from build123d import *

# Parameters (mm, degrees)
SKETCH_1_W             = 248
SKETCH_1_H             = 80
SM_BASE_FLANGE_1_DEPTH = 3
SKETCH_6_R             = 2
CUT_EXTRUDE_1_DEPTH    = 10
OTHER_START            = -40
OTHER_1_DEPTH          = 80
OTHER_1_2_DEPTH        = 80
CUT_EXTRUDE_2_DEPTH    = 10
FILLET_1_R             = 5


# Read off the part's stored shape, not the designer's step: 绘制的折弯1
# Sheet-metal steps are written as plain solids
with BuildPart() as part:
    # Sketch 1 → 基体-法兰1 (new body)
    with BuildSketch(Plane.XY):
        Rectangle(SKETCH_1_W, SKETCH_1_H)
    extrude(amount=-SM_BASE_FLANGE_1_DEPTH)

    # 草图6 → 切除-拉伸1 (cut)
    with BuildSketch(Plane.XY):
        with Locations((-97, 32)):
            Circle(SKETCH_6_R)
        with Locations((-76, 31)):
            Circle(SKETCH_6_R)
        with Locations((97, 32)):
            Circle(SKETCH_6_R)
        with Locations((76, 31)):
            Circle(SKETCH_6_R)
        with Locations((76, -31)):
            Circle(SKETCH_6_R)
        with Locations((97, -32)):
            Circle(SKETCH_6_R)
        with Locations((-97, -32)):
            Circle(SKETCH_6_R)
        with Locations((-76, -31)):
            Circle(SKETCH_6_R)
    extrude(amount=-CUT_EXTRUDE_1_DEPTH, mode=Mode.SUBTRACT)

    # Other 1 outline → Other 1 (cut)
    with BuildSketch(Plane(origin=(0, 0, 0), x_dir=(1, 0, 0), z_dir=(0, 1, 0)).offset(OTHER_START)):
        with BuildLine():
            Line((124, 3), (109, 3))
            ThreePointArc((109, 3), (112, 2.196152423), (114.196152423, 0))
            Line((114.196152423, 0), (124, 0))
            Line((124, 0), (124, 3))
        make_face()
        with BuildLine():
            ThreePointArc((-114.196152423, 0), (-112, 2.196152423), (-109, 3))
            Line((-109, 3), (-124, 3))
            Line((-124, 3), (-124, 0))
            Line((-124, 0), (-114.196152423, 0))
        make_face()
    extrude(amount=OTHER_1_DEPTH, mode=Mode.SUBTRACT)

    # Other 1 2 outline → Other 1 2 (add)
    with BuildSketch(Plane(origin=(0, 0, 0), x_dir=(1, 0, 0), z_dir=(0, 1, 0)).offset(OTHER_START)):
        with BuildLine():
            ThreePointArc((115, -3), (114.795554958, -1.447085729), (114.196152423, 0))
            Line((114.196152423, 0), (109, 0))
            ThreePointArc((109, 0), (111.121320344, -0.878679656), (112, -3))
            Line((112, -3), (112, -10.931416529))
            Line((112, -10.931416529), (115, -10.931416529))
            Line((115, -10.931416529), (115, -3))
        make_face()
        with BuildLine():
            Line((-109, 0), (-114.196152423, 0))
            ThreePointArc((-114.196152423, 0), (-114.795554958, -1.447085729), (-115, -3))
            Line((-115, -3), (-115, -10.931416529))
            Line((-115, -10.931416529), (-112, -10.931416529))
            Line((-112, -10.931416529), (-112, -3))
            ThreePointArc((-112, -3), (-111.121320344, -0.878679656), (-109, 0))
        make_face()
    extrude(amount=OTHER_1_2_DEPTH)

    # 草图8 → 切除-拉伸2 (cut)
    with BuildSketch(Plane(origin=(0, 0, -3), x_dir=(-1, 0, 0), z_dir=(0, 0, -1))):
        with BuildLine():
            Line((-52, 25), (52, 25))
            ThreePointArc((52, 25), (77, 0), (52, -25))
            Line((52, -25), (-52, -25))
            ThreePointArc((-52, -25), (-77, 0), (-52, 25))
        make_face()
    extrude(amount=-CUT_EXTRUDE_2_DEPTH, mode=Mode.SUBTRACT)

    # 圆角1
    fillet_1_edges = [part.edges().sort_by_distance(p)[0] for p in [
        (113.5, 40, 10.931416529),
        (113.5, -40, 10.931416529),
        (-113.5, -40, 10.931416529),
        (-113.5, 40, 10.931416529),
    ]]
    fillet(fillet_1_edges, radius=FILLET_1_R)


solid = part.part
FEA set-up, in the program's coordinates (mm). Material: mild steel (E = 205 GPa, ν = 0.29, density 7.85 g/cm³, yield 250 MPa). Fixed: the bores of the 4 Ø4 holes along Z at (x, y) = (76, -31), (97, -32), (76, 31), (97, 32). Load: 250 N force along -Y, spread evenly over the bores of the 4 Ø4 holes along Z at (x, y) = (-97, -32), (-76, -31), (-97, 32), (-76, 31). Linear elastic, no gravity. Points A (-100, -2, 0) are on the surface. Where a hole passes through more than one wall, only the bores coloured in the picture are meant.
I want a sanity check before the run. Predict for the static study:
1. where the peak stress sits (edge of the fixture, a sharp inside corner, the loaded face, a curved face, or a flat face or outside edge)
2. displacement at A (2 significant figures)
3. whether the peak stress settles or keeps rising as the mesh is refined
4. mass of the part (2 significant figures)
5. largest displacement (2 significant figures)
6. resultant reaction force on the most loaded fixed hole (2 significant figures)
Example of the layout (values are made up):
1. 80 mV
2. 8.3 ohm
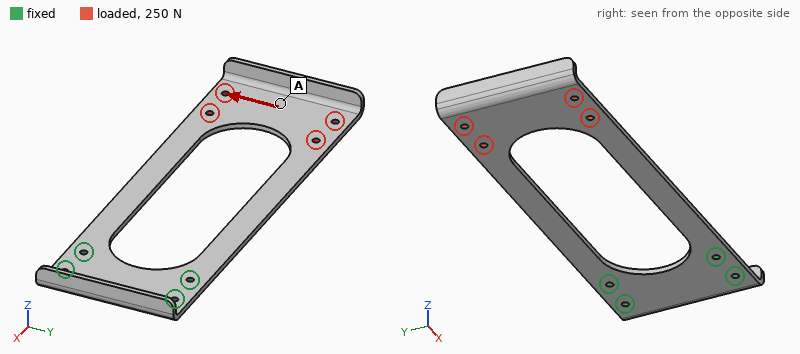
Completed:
1. edge of the fixture
2. 0.19 mm
3. keeps rising
4. 300 g
5. 0.19 mm
6. 540 N
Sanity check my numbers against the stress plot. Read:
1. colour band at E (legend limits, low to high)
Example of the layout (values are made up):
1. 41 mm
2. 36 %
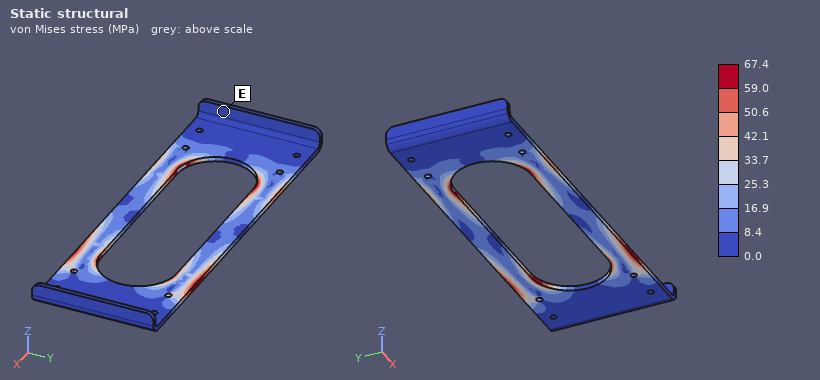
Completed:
1. 0.0 to 8.4 MPa
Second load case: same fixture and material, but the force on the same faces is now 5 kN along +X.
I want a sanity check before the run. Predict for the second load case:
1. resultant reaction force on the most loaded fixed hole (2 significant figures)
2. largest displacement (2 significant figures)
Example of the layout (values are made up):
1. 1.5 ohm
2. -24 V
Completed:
1. 2.1 kN
2. 44 µm
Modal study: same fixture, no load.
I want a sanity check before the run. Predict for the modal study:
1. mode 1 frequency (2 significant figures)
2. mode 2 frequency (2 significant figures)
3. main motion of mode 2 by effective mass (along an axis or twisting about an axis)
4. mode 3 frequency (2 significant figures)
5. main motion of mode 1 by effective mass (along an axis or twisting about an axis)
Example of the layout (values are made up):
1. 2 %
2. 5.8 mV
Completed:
1. 44 Hz
2. 220 Hz
3. twisting about X
4. 370 Hz
5. along Z
